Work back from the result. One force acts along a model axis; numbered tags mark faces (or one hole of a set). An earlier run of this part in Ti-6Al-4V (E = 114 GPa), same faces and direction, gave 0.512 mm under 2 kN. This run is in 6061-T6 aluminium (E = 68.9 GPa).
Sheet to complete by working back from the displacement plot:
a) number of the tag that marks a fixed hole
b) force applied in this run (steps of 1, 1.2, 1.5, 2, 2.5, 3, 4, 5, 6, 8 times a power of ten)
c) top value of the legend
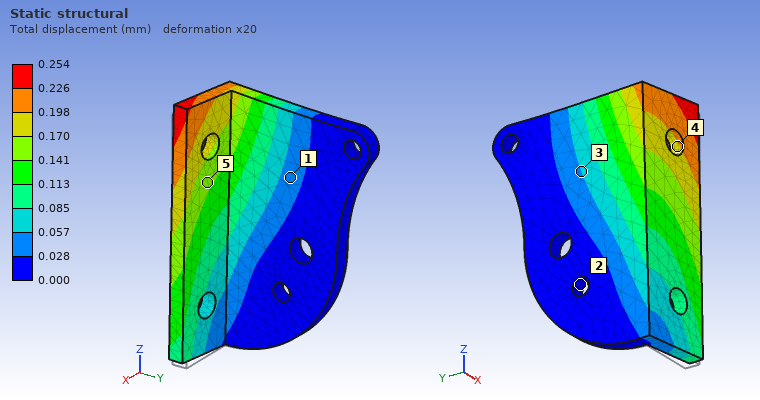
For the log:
2
600 N
0.254 mm
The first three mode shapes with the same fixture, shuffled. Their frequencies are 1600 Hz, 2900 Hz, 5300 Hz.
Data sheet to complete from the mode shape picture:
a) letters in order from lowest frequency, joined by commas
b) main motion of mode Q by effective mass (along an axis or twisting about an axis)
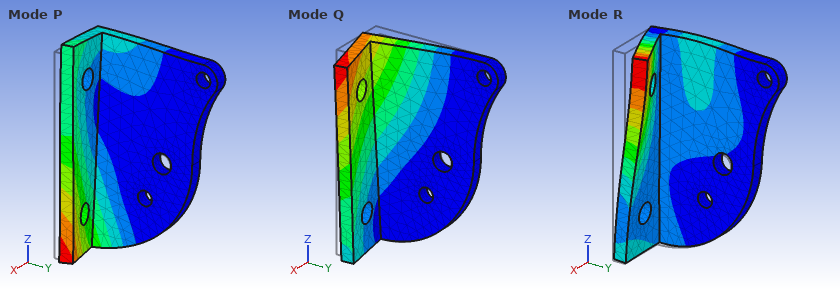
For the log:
Q, P, R
along X
